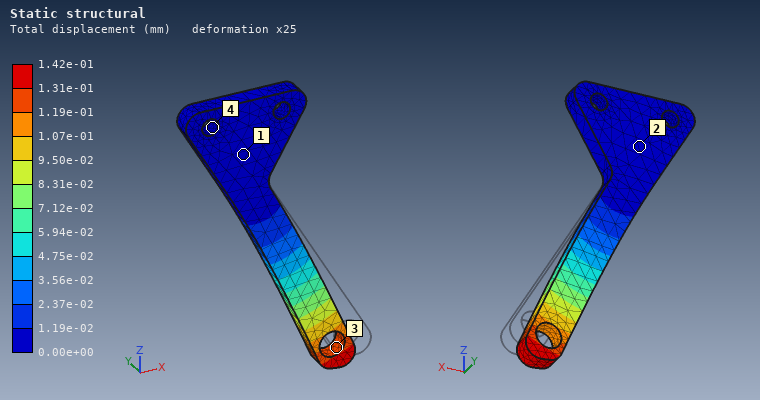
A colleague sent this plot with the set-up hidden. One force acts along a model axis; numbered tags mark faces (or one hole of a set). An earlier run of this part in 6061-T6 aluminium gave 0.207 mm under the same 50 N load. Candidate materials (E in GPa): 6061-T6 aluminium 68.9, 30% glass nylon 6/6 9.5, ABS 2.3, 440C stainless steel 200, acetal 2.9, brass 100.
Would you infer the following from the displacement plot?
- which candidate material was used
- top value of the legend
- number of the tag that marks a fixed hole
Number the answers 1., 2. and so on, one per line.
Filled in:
1. brass
2. 1.42e-01 mm
3. 4
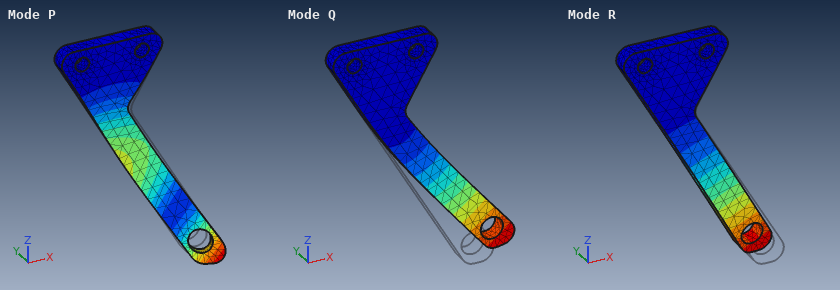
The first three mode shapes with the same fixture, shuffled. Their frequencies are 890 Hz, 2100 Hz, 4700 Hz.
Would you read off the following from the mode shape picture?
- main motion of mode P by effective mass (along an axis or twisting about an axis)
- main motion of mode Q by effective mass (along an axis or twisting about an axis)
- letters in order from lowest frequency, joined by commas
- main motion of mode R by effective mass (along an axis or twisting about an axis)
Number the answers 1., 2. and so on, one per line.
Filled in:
1. along Y
2. along X
3. R, Q, P
4. along Y
